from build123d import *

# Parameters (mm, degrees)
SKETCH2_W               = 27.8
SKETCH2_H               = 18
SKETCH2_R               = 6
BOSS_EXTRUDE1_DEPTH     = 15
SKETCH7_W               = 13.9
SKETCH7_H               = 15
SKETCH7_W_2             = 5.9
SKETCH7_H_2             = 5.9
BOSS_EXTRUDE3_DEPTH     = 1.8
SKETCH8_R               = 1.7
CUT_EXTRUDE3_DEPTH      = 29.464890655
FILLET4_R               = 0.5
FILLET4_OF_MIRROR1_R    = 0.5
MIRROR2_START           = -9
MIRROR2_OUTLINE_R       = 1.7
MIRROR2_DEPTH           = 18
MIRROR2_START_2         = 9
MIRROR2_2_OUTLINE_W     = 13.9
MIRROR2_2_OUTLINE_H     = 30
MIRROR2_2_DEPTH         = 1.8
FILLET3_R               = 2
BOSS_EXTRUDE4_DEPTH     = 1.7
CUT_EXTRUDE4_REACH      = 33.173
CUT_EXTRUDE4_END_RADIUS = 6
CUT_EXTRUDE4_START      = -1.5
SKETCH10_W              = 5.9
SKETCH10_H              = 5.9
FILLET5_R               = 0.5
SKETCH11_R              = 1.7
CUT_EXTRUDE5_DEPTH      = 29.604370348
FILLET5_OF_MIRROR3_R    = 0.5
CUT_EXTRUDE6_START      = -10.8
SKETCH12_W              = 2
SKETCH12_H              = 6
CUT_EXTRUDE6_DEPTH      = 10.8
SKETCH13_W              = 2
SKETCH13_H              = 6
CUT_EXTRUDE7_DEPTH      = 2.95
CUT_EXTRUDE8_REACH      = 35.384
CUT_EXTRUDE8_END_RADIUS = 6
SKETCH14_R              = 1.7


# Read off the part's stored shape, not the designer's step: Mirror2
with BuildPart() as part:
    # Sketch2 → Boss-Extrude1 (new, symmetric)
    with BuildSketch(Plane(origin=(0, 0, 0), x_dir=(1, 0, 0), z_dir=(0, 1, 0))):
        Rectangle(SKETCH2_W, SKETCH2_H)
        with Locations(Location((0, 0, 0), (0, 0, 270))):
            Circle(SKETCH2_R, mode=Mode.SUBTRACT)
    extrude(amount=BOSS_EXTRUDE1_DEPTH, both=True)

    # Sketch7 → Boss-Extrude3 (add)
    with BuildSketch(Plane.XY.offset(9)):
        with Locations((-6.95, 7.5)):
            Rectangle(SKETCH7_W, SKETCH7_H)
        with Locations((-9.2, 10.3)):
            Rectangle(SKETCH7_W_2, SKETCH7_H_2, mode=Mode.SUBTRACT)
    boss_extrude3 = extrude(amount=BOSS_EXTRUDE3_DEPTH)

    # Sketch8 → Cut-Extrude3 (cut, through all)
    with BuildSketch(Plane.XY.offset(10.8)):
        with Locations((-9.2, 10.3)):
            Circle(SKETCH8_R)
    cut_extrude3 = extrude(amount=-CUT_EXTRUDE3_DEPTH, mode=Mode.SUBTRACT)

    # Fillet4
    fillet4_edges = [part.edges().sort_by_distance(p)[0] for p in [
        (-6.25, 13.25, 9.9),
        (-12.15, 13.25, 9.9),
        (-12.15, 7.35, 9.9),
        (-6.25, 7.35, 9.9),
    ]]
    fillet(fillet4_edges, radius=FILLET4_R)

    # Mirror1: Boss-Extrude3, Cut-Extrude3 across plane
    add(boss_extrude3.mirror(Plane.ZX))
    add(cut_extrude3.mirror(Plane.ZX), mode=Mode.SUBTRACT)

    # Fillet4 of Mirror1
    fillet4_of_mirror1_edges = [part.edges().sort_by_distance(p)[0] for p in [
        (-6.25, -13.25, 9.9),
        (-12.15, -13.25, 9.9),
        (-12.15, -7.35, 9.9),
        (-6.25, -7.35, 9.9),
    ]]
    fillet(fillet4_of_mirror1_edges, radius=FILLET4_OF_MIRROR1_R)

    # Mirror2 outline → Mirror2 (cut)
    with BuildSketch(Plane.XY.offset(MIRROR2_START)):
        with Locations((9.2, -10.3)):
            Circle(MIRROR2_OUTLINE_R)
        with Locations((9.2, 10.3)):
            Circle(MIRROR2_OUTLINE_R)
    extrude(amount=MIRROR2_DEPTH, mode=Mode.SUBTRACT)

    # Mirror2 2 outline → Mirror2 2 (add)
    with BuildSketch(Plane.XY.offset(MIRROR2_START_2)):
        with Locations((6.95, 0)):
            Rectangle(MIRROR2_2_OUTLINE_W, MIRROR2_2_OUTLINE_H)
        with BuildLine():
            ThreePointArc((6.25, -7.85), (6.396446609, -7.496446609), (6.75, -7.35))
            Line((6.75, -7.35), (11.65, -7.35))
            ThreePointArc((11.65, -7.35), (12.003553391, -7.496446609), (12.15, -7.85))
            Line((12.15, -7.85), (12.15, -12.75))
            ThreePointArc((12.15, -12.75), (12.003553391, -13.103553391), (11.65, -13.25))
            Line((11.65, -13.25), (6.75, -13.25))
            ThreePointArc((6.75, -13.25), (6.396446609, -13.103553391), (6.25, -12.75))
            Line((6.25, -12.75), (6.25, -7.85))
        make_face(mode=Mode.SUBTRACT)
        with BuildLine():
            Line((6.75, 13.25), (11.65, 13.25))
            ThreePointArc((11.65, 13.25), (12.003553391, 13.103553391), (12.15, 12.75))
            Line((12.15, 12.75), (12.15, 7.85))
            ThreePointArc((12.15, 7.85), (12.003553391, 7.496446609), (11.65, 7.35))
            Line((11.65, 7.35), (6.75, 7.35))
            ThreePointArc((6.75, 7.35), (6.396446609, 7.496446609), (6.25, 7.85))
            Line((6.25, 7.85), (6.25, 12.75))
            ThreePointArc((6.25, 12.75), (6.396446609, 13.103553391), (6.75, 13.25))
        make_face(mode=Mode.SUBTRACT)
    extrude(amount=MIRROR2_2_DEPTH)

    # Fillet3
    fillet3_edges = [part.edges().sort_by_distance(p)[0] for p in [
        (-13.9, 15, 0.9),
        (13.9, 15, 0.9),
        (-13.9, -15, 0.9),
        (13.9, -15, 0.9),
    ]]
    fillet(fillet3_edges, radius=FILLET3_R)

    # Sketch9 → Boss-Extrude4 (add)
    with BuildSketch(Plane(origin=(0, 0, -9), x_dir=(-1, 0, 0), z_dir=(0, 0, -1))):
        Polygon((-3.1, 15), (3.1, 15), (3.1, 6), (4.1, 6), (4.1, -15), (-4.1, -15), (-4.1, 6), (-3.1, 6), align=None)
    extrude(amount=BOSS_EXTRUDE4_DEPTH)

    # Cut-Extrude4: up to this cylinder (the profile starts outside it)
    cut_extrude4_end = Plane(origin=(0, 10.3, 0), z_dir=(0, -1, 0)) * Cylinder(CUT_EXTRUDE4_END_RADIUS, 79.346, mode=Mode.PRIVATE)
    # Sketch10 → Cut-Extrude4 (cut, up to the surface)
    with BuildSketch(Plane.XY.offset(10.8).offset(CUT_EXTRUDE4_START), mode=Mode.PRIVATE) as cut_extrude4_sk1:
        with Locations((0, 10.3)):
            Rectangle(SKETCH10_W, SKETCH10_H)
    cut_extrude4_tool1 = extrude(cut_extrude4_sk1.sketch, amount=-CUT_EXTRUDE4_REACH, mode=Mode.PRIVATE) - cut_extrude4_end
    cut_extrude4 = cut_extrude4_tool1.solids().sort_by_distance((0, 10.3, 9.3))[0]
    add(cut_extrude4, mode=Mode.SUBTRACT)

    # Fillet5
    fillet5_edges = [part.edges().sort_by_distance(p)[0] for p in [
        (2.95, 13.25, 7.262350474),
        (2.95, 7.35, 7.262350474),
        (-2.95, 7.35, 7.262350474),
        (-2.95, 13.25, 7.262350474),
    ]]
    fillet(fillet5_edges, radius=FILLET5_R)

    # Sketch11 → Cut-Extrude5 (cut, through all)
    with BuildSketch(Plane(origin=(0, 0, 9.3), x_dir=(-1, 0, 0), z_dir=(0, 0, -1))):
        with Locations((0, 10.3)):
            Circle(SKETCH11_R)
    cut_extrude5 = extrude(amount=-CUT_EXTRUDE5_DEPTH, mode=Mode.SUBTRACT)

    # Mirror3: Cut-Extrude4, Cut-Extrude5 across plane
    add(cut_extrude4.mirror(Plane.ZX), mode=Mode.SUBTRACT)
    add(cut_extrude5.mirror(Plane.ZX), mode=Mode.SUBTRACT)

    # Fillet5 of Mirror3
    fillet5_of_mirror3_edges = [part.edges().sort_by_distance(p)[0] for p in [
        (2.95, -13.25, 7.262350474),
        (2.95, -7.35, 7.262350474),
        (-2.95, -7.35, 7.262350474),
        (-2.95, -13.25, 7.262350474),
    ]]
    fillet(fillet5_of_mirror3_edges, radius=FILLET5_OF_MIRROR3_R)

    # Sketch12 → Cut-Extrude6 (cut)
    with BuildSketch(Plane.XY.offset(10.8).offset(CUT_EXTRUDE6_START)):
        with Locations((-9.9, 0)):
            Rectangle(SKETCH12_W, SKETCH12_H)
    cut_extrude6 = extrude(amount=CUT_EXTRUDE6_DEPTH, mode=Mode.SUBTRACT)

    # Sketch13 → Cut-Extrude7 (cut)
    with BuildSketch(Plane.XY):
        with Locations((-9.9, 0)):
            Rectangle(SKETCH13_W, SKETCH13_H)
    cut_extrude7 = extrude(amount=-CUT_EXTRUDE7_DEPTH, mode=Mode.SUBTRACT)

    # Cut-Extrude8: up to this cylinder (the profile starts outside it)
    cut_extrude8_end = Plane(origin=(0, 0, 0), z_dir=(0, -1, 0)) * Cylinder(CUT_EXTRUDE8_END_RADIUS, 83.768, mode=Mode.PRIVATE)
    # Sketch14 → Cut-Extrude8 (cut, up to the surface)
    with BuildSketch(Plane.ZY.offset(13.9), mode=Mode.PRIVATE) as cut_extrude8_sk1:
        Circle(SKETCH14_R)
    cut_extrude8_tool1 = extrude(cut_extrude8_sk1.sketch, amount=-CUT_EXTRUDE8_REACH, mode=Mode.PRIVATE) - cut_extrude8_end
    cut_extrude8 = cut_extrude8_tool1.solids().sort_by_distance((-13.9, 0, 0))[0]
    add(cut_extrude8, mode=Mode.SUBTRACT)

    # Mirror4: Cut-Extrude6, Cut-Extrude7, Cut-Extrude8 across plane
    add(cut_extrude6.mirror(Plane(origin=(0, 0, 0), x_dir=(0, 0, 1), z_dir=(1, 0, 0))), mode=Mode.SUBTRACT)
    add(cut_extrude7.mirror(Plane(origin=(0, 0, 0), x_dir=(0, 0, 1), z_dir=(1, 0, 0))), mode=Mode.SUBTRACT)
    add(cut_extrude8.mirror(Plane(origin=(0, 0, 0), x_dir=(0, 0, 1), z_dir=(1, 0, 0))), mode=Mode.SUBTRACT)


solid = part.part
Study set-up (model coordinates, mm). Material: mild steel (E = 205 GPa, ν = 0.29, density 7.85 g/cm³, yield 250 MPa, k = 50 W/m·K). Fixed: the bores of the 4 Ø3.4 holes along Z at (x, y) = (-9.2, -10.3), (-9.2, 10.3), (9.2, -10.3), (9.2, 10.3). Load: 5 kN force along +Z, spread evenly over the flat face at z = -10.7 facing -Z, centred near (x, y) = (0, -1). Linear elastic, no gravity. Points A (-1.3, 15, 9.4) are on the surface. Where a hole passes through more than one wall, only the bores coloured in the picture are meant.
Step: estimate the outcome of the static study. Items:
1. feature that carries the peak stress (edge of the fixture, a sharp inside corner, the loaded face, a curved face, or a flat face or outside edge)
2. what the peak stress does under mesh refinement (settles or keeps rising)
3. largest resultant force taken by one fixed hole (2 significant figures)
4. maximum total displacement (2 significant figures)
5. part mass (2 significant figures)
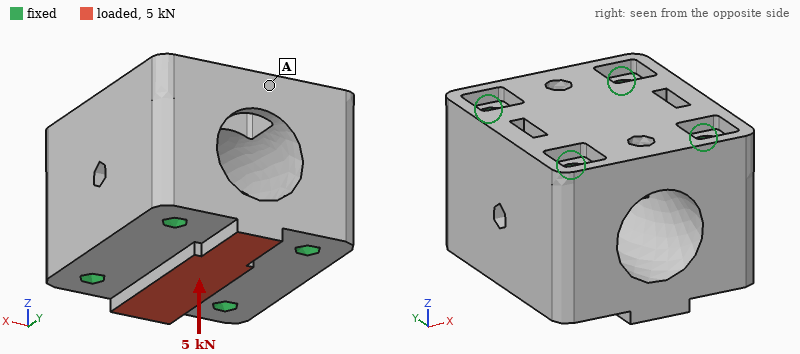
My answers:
edge of the fixture
keeps rising
1.6 kN
2.5 µm
93 g
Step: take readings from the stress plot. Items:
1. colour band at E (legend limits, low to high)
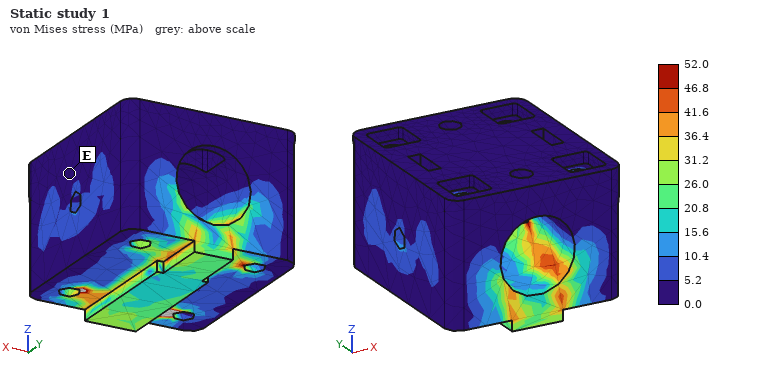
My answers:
0.0 to 5.2 MPa
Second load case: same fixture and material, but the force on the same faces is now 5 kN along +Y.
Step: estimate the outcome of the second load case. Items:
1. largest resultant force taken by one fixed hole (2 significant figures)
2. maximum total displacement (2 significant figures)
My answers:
1.5 kN
4.8 µm
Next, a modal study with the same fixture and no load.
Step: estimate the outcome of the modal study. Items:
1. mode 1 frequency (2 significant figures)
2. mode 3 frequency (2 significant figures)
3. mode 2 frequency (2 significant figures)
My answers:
63 kHz
70 kHz
63 kHz
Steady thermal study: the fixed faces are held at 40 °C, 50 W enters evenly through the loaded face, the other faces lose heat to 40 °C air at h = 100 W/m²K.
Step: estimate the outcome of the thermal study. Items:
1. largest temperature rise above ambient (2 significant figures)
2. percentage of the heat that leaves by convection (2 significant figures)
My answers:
37 K
4.2 %
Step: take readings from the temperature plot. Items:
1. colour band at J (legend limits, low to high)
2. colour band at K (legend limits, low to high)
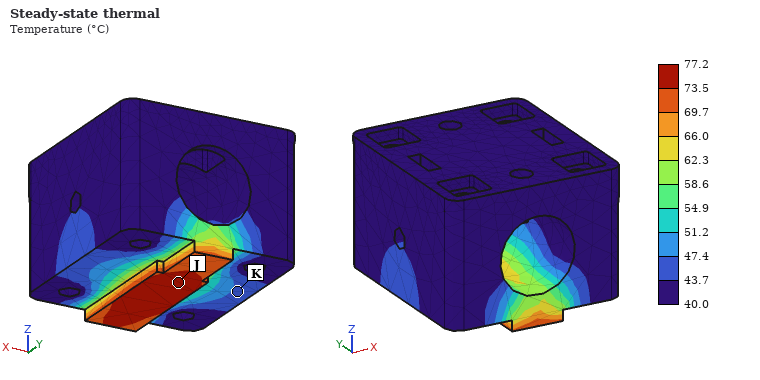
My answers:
73.5 to 77.2 °C
43.7 to 47.4 °C
